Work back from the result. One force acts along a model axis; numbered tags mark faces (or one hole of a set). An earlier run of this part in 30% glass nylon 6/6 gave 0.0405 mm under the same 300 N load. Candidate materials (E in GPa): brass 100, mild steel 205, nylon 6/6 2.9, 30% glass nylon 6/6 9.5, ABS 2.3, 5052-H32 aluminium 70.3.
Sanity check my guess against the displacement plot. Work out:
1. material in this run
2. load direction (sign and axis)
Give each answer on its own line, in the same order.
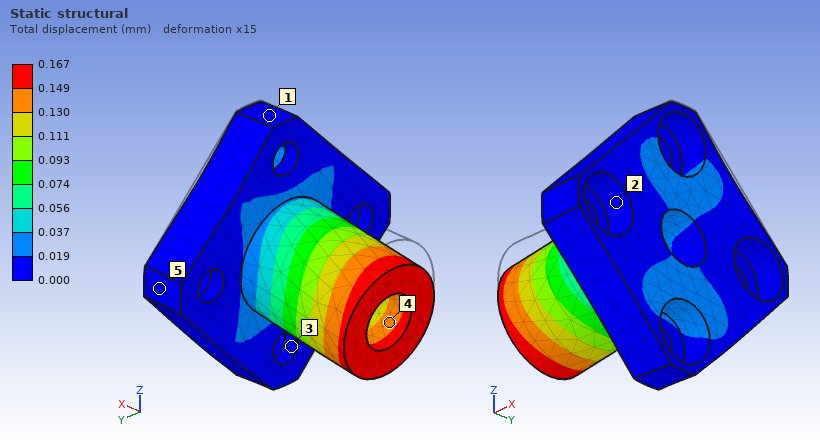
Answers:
ABS
-Z
